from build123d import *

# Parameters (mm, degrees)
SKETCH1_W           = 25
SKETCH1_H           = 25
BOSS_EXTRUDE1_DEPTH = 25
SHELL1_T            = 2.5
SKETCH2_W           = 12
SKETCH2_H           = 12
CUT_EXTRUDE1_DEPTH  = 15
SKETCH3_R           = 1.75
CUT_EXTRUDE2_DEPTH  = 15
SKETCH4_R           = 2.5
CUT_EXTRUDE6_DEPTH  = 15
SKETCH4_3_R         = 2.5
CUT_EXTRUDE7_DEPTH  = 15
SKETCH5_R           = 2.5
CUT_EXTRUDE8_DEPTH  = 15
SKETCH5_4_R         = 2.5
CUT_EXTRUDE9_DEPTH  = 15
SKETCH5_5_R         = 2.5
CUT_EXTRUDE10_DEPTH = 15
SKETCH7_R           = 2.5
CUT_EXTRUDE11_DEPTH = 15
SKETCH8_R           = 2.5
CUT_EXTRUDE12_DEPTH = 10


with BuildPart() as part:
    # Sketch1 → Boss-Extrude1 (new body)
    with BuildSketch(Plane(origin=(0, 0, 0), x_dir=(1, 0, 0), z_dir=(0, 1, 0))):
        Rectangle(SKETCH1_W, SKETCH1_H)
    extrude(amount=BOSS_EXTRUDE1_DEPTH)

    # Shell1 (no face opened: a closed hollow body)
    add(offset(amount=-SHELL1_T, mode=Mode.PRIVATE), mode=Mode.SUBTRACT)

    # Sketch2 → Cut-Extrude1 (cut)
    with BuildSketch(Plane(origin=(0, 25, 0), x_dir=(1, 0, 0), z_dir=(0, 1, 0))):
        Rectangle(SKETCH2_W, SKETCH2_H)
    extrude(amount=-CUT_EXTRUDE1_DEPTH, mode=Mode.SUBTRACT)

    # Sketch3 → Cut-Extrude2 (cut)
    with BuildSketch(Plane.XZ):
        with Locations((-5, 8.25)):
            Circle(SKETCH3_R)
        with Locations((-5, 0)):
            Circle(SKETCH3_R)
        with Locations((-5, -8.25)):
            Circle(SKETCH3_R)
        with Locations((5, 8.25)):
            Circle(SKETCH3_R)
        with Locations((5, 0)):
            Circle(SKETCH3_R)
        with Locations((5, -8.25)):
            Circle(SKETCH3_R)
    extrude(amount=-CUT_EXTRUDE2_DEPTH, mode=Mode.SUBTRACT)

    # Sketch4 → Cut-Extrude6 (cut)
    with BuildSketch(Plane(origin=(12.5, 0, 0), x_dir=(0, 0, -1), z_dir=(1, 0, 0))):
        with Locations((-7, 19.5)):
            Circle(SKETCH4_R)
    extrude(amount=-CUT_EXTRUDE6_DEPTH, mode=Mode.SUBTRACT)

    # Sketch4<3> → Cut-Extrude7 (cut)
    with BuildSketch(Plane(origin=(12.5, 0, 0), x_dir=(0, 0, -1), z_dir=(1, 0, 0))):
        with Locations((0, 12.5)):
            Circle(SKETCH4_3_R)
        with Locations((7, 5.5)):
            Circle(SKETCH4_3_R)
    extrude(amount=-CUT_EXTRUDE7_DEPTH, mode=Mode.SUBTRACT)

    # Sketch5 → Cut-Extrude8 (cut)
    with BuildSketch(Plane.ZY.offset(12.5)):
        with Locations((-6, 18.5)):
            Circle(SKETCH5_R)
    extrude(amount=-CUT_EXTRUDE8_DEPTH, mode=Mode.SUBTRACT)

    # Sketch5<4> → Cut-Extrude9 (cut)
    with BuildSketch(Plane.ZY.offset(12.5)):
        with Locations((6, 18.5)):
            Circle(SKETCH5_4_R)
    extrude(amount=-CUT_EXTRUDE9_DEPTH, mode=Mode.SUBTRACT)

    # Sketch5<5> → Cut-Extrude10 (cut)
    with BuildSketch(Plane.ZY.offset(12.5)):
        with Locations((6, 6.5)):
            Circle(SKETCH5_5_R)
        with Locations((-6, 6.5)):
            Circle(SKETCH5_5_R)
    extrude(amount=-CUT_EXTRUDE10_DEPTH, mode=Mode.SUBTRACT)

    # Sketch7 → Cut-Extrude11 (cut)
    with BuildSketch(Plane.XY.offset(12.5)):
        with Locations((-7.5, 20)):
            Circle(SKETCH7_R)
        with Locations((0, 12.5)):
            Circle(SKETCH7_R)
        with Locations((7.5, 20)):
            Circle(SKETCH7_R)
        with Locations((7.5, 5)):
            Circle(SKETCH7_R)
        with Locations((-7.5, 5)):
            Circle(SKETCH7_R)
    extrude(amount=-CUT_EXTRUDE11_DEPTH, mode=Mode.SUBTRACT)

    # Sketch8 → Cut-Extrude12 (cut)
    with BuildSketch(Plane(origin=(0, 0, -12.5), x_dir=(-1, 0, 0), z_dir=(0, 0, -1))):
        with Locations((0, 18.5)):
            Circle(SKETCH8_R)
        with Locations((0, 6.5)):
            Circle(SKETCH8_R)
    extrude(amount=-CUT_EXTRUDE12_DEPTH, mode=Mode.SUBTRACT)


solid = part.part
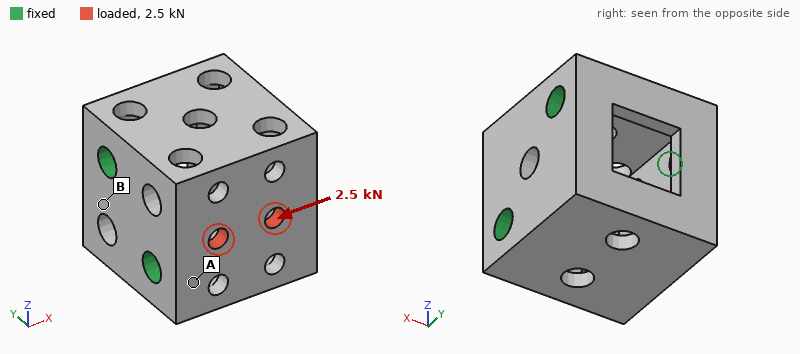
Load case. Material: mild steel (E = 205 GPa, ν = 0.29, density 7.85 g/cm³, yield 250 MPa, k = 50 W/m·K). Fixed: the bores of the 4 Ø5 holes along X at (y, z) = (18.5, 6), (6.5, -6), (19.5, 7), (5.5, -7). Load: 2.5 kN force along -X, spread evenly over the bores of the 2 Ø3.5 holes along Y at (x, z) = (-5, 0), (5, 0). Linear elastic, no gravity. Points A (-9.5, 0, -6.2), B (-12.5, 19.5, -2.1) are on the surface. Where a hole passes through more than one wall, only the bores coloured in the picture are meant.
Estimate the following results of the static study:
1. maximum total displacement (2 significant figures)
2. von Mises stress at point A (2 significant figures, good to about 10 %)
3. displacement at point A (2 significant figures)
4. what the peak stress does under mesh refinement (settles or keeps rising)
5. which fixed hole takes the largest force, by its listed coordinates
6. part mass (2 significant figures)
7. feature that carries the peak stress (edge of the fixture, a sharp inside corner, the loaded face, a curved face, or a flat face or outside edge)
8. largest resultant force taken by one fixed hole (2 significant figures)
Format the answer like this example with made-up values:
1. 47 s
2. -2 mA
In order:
1. 6.5 µm
2. 45 MPa
3. 3.3 µm
4. keeps rising
5. (5.5, -7)
6. 51 g
7. edge of the fixture
8. 1.2 kN
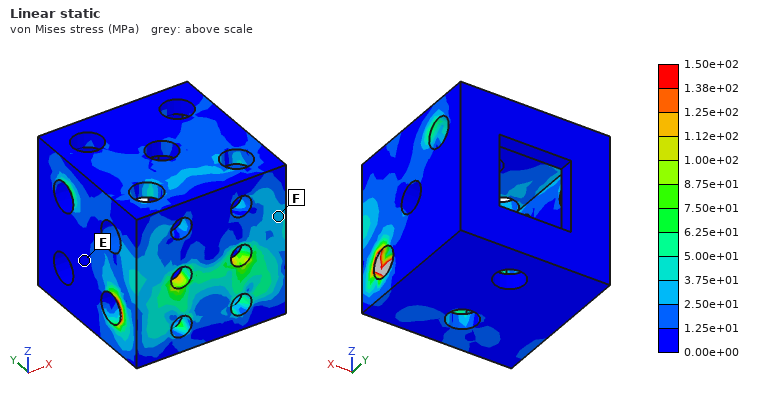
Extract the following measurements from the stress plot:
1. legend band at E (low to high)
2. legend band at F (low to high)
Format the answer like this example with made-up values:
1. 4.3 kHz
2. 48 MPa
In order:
1. 0.00e+00 to 1.25e+01 MPa
2. 2.50e+01 to 3.75e+01 MPa
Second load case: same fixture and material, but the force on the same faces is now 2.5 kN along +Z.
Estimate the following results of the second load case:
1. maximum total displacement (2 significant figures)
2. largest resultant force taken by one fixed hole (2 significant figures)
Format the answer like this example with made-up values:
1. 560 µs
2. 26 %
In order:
1. 5.2 µm
2. 1.3 kN
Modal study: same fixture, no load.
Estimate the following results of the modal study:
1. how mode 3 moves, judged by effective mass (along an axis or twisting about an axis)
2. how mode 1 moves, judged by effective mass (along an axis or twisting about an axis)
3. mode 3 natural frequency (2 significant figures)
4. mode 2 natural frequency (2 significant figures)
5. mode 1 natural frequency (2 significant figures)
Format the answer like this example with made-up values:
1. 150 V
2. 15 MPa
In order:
1. along Z
2. along X
3. 28 kHz
4. 26 kHz
5. 24 kHz
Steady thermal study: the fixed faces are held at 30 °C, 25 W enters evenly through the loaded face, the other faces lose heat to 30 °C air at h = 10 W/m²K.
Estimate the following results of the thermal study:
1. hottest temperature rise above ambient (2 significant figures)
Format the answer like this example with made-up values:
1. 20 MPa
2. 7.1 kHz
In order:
1. 66 K
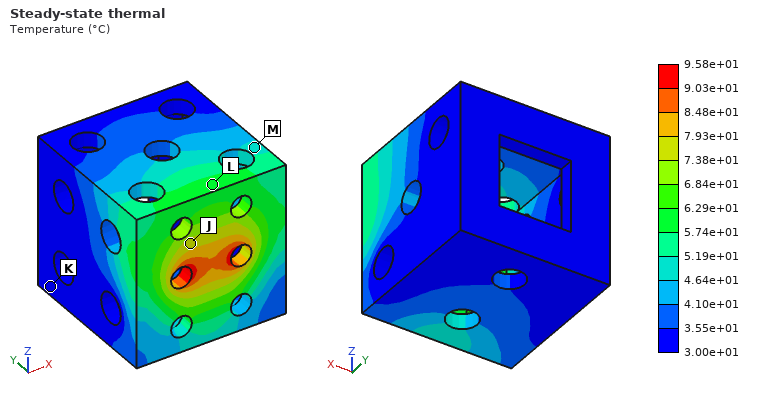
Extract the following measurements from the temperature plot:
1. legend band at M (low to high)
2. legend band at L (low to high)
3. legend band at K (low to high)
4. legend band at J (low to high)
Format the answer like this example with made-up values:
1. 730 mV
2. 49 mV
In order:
1. 4.64e+01 to 5.19e+01 °C
2. 5.74e+01 to 6.29e+01 °C
3. 3.00e+01 to 3.55e+01 °C
4. 7.38e+01 to 7.93e+01 °C
